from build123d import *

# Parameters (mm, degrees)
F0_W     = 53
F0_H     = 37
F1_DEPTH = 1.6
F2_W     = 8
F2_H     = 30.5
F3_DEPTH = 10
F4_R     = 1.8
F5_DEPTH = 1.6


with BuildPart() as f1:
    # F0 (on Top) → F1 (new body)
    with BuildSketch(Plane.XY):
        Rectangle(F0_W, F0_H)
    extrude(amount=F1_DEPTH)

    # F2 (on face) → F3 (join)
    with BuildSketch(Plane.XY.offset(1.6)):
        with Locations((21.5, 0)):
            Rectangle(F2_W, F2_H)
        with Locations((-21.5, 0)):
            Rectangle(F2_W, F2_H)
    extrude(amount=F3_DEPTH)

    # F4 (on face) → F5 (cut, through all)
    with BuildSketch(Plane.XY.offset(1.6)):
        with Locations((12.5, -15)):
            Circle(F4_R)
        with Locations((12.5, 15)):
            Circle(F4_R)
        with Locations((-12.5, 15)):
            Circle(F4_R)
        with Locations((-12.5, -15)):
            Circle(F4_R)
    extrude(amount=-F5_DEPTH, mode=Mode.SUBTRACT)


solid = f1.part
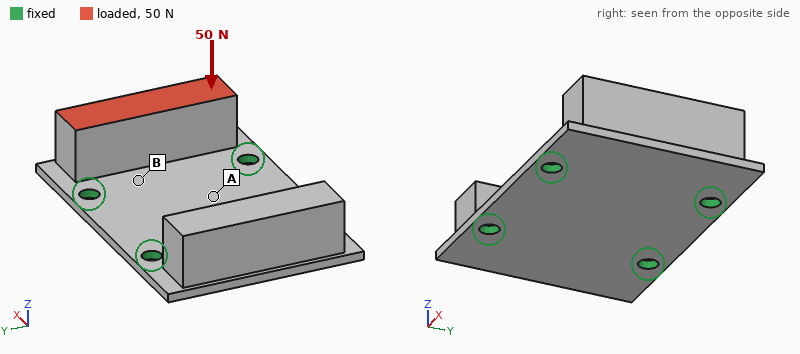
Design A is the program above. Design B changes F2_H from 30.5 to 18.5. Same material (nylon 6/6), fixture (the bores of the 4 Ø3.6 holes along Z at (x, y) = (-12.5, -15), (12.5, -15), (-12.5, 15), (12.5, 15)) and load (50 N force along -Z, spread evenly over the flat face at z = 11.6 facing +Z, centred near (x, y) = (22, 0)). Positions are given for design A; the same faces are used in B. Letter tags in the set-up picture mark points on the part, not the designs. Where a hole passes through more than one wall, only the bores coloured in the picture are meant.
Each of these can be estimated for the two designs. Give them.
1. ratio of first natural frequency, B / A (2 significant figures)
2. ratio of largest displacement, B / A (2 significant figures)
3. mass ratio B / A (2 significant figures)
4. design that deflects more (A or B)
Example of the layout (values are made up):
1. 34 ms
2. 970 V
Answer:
1. 1.1
2. 1.3
3. 0.76
4. B
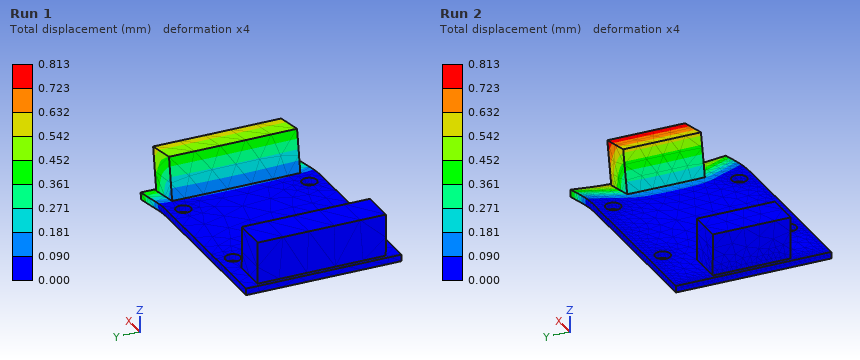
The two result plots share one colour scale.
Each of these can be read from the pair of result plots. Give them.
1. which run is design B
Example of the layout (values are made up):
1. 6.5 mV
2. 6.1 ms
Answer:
1. Run 2
